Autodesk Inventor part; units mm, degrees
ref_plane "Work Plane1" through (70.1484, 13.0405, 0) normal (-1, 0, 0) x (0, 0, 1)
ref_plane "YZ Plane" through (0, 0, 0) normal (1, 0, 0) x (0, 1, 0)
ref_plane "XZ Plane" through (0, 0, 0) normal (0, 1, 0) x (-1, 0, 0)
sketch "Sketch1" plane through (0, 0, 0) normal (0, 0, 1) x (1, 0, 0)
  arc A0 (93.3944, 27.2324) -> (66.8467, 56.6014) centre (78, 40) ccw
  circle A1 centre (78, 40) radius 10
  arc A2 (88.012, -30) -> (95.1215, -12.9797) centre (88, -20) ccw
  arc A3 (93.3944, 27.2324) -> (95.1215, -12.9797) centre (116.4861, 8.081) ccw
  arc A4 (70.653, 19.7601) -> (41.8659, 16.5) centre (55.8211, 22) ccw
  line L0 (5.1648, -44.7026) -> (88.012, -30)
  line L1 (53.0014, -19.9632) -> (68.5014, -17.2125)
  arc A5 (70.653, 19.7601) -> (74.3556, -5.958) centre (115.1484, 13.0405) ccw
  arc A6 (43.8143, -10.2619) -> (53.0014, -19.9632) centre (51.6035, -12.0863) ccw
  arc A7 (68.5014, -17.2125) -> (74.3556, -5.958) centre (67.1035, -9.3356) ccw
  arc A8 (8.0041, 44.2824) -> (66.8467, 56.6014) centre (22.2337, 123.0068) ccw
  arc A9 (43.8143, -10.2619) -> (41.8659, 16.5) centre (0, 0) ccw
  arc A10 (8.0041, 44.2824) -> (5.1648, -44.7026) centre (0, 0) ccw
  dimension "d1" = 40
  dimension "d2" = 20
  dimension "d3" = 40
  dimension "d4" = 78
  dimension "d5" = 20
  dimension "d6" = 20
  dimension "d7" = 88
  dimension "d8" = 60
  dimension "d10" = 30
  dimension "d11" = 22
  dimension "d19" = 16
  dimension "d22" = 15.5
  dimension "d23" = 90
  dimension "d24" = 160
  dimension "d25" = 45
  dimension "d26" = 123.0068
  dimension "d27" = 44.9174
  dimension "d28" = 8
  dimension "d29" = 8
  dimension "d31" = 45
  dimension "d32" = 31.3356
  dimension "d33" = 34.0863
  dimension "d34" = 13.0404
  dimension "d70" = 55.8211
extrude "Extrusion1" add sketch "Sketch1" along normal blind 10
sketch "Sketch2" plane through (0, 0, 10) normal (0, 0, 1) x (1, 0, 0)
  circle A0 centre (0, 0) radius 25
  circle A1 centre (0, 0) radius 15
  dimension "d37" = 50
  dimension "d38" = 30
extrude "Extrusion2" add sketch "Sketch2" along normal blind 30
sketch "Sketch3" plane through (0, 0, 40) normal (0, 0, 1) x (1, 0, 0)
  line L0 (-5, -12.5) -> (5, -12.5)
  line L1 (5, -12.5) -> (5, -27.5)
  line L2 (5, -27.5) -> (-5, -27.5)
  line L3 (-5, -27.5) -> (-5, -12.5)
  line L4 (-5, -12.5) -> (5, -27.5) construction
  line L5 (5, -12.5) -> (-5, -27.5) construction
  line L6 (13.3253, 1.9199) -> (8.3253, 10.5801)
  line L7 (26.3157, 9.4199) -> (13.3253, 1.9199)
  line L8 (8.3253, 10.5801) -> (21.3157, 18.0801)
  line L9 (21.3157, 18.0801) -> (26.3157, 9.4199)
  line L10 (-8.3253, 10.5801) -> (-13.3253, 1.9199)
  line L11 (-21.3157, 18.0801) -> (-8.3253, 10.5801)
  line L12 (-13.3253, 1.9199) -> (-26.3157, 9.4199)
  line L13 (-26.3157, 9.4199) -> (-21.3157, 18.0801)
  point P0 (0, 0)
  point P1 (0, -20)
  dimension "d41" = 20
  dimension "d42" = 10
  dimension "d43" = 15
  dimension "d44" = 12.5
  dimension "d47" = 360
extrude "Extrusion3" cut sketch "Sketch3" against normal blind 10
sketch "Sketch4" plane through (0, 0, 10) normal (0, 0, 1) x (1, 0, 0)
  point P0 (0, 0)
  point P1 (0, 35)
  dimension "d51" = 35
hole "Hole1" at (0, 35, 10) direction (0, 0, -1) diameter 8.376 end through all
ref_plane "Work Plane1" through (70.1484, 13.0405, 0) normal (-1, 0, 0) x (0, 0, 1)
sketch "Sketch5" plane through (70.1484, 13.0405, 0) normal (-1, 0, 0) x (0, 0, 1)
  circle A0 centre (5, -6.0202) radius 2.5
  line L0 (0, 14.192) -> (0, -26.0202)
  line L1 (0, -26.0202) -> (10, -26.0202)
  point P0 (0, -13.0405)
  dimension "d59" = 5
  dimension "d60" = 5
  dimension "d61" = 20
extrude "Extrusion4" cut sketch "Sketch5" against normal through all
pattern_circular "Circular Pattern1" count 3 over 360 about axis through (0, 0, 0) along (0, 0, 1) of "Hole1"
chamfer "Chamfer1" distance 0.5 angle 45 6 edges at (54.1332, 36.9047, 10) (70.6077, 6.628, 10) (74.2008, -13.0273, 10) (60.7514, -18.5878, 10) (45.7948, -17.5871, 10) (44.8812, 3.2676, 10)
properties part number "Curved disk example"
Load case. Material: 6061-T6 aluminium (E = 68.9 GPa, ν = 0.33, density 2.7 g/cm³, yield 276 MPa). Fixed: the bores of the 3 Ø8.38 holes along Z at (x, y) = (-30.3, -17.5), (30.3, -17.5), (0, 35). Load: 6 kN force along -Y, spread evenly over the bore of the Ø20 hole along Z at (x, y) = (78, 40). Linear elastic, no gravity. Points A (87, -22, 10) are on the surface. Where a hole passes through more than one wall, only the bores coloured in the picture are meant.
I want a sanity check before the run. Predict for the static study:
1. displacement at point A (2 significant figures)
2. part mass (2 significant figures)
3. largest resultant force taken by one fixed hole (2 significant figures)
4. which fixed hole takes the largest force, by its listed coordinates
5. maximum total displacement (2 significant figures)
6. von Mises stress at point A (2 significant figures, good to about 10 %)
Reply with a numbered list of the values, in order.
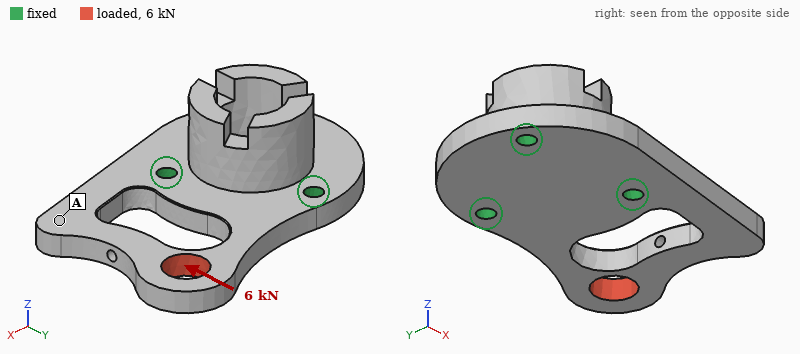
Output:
1. 0.17 mm
2. 340 g
3. 7.2 kN
4. (30.3, -17.5)
5. 0.23 mm
6. 24 MPa
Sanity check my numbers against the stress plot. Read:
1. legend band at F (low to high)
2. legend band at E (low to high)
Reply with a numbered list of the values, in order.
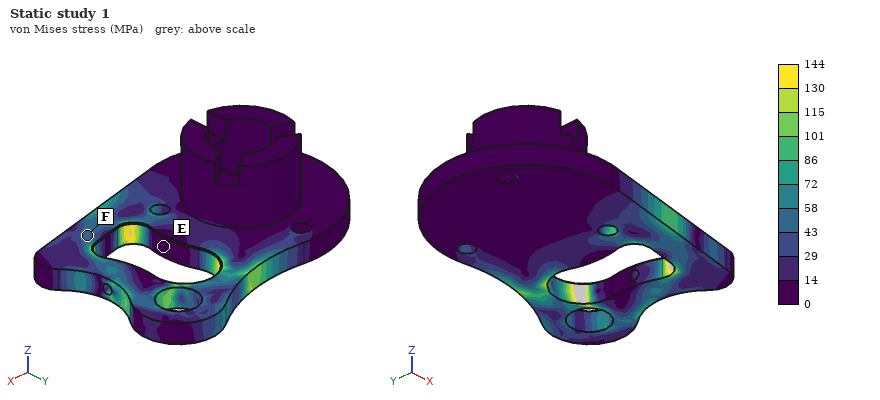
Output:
1. 43 to 58 MPa
2. 0 to 14 MPa
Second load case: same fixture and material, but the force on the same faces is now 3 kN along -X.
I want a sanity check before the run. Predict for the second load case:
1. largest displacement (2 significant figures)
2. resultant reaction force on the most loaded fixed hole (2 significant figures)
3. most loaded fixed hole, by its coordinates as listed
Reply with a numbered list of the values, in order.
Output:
1. 52 µm
2. 2.7 kN
3. (0, 35)
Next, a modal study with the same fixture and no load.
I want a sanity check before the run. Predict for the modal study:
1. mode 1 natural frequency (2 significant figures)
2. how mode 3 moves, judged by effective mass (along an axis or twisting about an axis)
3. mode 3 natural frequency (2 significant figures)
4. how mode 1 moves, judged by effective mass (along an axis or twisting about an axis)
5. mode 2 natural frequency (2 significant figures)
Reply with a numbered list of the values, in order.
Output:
1. 1200 Hz
2. along Y
3. 3900 Hz
4. along Z
5. 2300 Hz
